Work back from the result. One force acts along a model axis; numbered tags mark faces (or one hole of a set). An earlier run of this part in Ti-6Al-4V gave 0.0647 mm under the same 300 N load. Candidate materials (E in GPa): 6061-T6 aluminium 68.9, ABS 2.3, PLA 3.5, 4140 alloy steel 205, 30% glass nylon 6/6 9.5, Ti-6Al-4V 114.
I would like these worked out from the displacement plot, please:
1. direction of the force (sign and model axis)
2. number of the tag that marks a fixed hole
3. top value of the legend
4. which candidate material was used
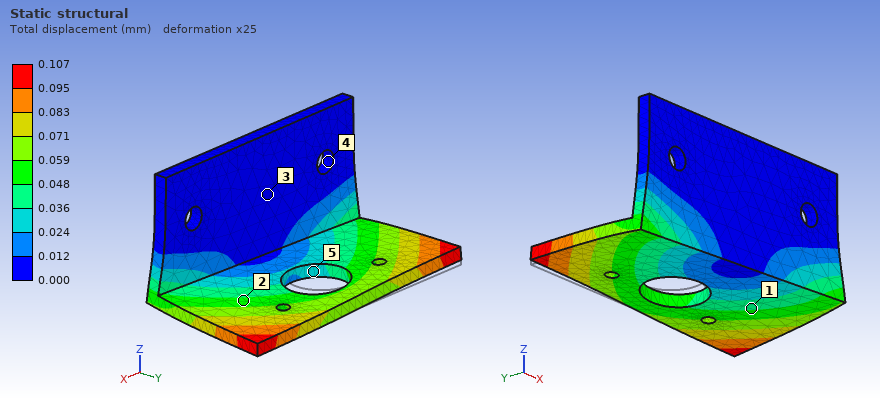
+X
4
0.107 mm
6061-T6 aluminium
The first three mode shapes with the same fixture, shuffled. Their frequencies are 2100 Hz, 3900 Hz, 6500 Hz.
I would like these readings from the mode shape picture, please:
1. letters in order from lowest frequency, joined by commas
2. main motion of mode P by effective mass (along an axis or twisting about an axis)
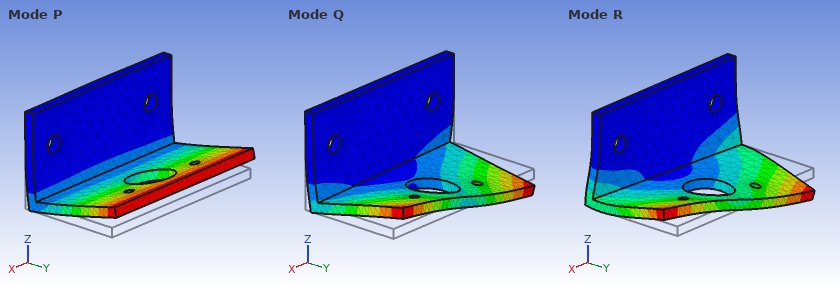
P, Q, R
along Z
